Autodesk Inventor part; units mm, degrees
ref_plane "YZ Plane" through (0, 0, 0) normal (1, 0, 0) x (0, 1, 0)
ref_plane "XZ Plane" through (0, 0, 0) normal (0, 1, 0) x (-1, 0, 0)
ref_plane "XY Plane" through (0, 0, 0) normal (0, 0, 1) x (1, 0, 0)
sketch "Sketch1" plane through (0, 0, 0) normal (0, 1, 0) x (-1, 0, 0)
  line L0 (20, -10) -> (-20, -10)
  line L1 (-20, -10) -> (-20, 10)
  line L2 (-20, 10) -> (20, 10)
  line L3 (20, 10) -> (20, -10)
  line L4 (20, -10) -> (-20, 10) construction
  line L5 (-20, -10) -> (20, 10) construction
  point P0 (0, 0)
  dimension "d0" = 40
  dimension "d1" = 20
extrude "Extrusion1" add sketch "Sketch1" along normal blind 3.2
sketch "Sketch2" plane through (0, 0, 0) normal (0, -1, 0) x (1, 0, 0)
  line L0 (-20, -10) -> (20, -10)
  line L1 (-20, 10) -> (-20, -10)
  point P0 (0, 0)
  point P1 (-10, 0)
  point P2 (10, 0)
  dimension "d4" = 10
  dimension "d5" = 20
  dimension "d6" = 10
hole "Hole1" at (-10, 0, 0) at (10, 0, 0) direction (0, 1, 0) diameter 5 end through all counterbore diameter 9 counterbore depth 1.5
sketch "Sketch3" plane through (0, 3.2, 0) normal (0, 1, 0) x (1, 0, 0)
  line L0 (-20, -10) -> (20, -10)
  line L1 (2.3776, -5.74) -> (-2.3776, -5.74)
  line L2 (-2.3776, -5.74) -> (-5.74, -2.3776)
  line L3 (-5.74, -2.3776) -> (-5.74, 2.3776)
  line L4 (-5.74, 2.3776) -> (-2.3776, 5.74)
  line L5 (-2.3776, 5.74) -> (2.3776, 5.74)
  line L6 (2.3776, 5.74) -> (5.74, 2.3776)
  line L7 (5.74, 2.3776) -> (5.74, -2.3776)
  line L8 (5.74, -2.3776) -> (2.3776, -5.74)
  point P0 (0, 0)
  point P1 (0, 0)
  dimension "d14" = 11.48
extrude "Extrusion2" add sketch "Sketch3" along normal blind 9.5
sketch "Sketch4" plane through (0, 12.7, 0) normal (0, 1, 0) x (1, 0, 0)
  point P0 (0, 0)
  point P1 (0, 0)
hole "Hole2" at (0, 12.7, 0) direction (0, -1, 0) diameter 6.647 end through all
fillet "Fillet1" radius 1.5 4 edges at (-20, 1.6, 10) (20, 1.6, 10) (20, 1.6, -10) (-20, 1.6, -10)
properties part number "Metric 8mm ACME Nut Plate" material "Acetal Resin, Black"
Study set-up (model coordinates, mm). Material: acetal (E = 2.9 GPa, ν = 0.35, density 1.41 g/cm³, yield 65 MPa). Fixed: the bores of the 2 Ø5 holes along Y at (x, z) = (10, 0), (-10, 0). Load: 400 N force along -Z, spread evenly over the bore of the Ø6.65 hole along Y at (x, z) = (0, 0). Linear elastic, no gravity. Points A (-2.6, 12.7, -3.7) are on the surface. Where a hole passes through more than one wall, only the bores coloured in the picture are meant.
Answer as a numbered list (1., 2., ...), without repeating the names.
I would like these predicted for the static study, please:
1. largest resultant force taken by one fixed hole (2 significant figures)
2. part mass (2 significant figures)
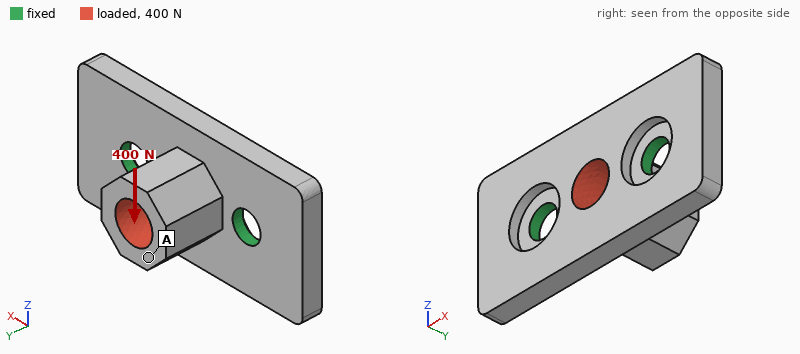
1. 200 N
2. 4.1 g
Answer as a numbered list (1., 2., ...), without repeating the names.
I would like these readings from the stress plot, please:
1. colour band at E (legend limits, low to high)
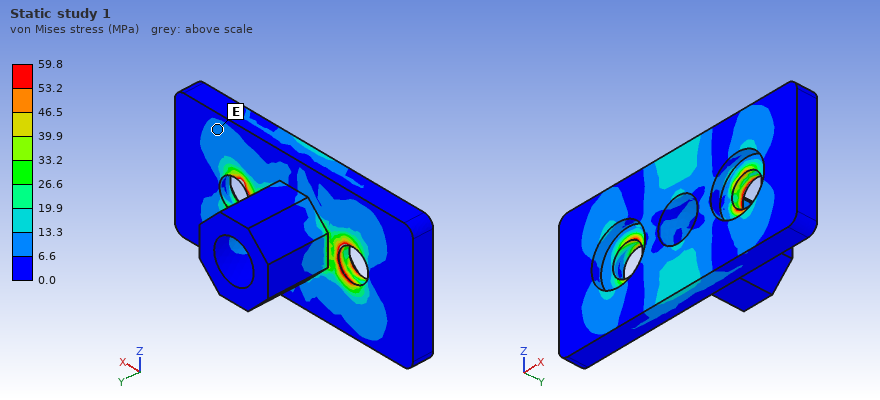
1. 6.6 to 13.3 MPa
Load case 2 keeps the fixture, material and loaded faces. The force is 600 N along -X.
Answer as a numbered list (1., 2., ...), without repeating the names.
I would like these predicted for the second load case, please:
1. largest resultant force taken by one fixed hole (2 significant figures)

1. 340 N
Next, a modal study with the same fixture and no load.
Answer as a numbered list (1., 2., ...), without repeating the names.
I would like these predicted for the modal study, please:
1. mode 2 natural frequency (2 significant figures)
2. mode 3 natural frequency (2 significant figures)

1. 5000 Hz
2. 5100 Hz
